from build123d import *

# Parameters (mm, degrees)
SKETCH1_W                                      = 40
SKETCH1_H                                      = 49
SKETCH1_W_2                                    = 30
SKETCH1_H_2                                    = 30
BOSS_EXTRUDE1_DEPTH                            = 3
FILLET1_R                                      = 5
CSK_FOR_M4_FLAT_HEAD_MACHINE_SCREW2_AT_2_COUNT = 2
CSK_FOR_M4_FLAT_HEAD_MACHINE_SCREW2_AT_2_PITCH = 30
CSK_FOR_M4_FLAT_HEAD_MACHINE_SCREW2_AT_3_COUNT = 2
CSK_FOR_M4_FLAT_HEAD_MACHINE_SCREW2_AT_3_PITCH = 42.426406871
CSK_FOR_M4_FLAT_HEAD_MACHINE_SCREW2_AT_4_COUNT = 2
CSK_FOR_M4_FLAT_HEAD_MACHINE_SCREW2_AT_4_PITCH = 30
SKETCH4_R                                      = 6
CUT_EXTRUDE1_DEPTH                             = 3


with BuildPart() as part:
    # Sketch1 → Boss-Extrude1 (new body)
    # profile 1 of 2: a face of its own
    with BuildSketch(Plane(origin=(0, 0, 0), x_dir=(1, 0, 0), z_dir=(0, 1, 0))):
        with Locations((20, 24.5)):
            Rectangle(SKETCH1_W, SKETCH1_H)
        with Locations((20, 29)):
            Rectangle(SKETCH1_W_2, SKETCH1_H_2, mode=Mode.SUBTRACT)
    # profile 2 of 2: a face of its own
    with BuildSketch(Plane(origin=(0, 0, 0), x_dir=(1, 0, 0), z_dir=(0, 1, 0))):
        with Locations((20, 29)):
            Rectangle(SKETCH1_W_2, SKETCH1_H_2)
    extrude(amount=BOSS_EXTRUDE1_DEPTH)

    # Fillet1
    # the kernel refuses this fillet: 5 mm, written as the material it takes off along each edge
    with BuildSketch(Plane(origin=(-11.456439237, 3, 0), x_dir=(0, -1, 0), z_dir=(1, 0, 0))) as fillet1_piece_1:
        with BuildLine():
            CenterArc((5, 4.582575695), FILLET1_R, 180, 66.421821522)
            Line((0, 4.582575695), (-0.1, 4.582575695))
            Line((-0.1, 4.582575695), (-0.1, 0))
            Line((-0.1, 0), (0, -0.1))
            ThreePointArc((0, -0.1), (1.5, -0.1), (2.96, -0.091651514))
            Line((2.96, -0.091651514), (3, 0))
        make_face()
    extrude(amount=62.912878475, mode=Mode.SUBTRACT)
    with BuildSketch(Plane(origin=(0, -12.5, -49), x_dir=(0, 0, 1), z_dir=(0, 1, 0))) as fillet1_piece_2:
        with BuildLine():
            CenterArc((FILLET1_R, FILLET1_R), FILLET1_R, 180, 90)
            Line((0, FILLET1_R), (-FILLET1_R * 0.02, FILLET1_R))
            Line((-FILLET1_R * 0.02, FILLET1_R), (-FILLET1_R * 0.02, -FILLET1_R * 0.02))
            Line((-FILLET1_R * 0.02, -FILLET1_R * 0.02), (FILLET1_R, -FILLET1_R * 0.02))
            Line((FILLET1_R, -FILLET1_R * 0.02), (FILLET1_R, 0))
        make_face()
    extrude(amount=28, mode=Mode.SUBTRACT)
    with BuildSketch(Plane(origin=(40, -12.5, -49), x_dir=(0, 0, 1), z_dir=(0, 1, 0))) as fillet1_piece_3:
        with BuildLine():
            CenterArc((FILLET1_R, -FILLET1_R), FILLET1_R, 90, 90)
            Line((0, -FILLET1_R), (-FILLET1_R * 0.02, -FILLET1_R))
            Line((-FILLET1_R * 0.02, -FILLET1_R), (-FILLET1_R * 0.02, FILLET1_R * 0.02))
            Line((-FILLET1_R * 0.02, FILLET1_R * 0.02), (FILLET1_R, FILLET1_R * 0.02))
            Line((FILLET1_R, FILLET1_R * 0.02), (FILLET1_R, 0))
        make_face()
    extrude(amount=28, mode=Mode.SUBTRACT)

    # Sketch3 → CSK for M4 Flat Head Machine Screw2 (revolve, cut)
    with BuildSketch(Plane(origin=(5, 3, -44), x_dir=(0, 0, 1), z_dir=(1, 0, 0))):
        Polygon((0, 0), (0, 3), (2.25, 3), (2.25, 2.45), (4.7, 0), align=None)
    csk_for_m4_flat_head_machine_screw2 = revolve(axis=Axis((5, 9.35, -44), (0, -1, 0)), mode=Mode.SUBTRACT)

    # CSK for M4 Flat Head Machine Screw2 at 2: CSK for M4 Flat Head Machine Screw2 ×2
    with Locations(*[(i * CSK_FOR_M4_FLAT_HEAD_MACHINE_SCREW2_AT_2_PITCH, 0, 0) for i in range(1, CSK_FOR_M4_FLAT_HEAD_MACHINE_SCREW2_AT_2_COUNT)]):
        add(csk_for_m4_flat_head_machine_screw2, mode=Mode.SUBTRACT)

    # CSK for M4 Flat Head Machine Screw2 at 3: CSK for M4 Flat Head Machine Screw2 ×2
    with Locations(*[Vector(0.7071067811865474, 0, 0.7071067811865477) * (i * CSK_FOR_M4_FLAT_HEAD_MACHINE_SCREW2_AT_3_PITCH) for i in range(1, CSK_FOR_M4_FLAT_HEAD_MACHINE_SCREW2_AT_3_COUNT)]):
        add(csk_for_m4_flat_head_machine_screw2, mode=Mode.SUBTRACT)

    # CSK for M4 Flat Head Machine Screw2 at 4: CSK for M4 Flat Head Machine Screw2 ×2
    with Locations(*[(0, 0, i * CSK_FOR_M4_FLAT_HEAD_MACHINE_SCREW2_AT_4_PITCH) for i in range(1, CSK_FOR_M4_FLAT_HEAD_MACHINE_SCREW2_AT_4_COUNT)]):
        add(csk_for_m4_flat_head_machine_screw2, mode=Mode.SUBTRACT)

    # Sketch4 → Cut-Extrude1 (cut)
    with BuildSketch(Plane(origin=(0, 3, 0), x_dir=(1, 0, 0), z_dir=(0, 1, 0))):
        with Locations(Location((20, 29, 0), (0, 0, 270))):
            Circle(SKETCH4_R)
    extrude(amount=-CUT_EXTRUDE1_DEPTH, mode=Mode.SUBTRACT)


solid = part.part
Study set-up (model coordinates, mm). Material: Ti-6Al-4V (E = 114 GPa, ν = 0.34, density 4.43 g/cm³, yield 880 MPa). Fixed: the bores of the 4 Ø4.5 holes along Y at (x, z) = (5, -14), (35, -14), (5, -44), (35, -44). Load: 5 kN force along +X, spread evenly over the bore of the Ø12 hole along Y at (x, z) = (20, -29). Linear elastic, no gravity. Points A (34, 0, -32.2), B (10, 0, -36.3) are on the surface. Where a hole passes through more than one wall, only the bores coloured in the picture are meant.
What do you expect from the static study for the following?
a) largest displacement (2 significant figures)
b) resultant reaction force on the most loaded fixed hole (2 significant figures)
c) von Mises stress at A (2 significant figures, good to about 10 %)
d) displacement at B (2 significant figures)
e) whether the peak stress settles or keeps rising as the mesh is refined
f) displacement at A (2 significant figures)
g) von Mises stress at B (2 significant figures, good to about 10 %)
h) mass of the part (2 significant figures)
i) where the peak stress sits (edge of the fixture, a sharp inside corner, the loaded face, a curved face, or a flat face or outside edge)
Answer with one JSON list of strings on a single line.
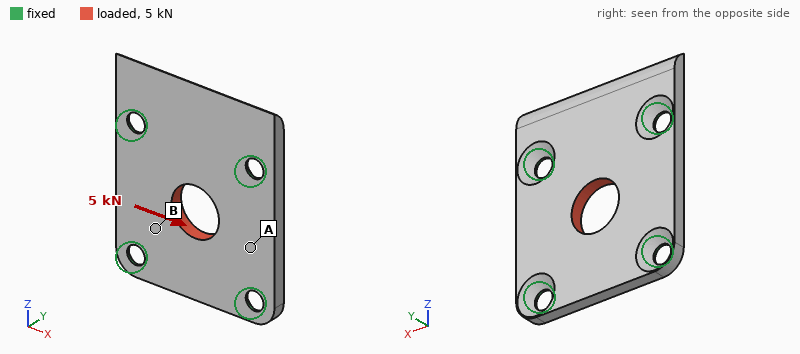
["13 µm", "1.3 kN", "29 MPa", "8.4 µm", "keeps rising", "9.0 µm", "51 MPa", "22 g", "edge of the fixture"]
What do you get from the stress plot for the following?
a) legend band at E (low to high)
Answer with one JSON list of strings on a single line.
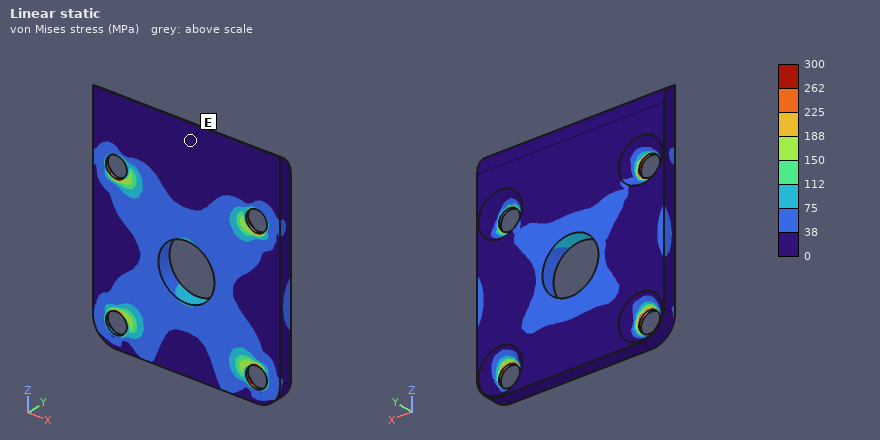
["0 to 38 MPa"]
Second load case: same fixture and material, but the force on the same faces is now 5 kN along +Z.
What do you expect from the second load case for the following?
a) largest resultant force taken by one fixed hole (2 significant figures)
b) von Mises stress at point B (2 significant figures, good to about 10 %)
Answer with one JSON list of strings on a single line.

["1.3 kN", "48 MPa"]
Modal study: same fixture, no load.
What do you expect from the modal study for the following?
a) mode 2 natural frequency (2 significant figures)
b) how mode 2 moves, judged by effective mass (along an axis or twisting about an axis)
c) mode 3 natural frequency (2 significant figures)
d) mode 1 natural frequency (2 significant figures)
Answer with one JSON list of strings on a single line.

["11 kHz", "along Y", "13 kHz", "8000 Hz"]
